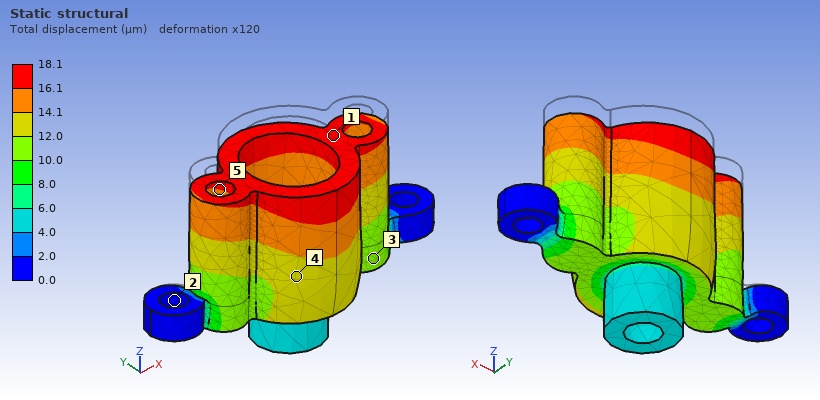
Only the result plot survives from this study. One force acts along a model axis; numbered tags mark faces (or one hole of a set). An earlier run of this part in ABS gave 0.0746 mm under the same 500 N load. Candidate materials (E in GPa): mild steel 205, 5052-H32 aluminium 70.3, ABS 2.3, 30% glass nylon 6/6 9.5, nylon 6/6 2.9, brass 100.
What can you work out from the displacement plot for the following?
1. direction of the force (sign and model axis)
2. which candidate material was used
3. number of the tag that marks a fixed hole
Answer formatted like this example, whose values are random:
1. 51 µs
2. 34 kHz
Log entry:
1. -Z
2. 30% glass nylon 6/6
3. 2
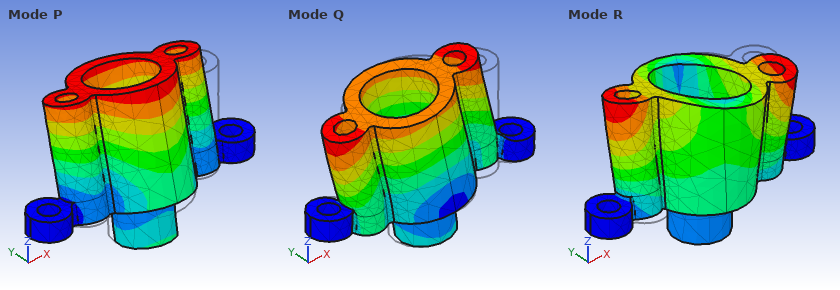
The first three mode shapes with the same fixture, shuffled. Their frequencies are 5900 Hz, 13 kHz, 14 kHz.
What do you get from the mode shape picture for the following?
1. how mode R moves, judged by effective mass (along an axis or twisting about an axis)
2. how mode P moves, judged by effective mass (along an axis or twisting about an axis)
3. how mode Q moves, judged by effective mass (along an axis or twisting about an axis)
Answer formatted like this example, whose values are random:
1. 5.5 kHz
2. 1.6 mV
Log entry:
1. twisting about Z
2. along Y
3. along X
